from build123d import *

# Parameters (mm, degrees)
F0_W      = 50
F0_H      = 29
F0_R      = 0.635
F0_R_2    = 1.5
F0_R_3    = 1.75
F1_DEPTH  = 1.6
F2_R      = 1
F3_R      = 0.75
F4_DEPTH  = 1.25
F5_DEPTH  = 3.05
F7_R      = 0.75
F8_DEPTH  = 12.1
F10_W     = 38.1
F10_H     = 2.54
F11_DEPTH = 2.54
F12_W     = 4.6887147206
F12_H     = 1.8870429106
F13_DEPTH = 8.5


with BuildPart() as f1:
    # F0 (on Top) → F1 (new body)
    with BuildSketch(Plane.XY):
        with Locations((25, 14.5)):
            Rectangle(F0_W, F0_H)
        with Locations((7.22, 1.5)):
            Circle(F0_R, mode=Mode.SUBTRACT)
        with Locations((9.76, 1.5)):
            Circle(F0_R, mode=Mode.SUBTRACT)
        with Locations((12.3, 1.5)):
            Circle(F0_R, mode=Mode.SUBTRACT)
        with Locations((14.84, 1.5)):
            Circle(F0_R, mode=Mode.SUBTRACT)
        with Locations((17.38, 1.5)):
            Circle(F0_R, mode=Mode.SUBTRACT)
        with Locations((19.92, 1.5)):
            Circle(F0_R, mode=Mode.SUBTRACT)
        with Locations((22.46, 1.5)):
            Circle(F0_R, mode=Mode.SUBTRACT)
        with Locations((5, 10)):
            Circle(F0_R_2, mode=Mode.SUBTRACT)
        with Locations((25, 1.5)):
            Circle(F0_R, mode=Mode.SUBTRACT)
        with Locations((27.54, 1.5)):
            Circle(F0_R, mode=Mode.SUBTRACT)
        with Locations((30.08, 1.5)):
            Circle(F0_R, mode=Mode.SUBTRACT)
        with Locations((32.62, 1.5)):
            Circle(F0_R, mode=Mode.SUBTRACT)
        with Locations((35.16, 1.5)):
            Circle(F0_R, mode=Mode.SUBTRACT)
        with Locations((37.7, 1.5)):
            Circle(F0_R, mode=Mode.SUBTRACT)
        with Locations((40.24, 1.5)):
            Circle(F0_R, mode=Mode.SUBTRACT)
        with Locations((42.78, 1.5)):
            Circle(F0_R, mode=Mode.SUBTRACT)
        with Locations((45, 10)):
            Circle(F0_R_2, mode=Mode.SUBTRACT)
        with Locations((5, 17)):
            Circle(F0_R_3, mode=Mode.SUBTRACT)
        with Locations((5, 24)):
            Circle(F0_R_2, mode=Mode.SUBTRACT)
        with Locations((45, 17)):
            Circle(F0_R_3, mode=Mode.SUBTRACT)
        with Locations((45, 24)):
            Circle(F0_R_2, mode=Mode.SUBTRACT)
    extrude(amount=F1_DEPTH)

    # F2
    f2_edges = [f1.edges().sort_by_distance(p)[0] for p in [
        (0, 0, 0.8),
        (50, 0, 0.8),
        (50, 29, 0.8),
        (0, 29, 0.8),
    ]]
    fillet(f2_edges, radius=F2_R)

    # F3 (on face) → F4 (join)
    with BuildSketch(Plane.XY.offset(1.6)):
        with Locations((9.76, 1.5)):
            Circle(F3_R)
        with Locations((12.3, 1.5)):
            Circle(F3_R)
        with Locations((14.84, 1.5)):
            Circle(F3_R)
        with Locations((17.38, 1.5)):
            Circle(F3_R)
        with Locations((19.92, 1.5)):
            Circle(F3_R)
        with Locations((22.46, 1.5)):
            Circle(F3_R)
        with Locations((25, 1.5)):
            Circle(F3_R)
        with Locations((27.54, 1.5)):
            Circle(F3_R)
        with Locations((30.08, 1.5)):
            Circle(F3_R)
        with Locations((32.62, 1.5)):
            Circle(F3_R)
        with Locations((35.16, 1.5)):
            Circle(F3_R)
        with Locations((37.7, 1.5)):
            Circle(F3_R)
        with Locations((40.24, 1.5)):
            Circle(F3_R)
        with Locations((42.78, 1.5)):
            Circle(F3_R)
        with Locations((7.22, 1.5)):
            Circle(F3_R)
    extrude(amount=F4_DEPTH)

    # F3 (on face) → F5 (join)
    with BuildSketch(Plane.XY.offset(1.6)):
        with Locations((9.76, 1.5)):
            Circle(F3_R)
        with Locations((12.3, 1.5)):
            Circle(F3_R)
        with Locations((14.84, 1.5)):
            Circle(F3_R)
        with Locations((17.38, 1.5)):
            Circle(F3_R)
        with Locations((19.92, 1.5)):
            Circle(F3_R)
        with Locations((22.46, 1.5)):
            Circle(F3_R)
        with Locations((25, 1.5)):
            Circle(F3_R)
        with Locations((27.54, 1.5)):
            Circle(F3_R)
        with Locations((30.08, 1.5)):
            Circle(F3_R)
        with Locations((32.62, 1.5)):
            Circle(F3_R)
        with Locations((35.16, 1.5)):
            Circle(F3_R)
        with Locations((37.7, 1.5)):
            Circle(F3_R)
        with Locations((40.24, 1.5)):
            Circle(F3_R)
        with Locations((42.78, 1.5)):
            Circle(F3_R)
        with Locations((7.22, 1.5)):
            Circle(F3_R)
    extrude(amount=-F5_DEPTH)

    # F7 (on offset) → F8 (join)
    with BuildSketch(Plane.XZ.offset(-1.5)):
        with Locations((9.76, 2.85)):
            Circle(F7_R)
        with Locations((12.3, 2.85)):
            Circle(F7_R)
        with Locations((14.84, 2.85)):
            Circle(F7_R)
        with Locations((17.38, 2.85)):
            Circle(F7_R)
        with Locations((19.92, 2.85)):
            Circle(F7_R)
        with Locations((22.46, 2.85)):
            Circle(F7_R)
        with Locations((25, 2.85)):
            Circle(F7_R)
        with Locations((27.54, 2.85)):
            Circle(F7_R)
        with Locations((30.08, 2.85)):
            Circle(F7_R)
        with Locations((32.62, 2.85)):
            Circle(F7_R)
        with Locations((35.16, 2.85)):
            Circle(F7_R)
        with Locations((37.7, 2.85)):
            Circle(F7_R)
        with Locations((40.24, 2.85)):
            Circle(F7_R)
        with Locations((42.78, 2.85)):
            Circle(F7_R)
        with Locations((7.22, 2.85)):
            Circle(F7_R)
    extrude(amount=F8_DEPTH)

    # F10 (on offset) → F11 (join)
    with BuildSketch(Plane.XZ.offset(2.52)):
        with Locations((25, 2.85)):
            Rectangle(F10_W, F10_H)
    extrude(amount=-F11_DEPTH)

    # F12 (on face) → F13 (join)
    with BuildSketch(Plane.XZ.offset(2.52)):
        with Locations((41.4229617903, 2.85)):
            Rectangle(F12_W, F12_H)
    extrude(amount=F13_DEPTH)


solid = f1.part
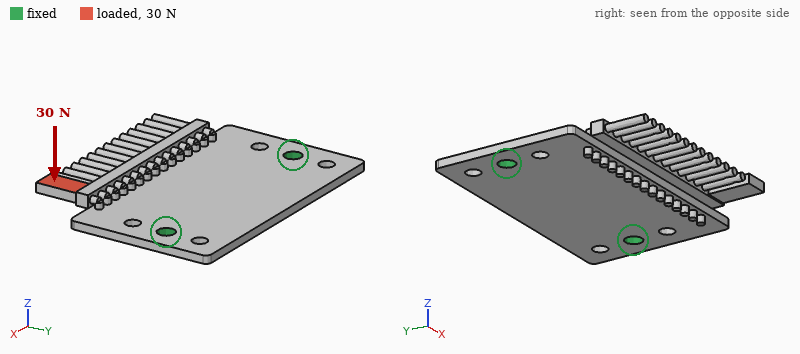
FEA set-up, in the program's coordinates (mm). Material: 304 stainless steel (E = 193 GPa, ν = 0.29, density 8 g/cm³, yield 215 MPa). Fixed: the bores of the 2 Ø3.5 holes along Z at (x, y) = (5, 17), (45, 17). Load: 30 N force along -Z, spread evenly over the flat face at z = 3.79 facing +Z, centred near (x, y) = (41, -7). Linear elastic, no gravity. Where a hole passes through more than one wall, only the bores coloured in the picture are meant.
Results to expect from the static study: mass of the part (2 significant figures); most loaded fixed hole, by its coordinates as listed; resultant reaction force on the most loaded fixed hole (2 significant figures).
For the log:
23 g
(45, 17)
28 N
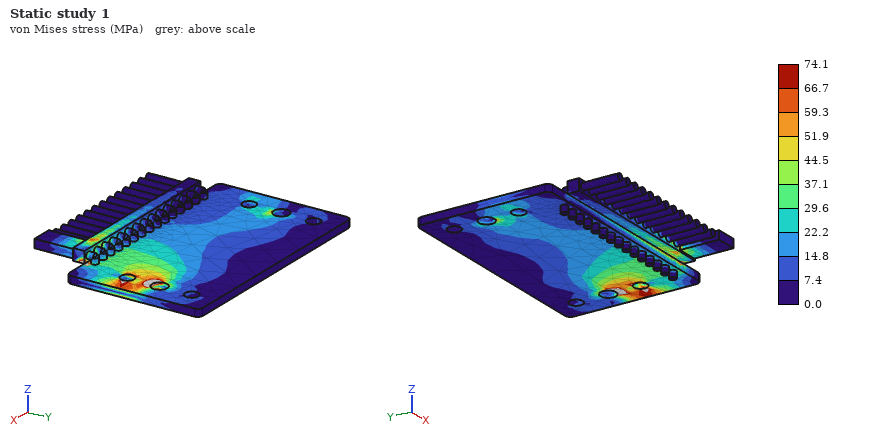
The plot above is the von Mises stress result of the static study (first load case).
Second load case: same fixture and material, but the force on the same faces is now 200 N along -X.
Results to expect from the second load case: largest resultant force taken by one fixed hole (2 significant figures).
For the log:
160 N
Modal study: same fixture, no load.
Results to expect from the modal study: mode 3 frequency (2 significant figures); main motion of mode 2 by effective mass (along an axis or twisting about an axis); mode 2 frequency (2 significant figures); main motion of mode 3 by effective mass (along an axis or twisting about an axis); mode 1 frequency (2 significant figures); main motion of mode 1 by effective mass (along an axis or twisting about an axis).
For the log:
4700 Hz
twisting about Y
3600 Hz
along Z
1800 Hz
along Z
